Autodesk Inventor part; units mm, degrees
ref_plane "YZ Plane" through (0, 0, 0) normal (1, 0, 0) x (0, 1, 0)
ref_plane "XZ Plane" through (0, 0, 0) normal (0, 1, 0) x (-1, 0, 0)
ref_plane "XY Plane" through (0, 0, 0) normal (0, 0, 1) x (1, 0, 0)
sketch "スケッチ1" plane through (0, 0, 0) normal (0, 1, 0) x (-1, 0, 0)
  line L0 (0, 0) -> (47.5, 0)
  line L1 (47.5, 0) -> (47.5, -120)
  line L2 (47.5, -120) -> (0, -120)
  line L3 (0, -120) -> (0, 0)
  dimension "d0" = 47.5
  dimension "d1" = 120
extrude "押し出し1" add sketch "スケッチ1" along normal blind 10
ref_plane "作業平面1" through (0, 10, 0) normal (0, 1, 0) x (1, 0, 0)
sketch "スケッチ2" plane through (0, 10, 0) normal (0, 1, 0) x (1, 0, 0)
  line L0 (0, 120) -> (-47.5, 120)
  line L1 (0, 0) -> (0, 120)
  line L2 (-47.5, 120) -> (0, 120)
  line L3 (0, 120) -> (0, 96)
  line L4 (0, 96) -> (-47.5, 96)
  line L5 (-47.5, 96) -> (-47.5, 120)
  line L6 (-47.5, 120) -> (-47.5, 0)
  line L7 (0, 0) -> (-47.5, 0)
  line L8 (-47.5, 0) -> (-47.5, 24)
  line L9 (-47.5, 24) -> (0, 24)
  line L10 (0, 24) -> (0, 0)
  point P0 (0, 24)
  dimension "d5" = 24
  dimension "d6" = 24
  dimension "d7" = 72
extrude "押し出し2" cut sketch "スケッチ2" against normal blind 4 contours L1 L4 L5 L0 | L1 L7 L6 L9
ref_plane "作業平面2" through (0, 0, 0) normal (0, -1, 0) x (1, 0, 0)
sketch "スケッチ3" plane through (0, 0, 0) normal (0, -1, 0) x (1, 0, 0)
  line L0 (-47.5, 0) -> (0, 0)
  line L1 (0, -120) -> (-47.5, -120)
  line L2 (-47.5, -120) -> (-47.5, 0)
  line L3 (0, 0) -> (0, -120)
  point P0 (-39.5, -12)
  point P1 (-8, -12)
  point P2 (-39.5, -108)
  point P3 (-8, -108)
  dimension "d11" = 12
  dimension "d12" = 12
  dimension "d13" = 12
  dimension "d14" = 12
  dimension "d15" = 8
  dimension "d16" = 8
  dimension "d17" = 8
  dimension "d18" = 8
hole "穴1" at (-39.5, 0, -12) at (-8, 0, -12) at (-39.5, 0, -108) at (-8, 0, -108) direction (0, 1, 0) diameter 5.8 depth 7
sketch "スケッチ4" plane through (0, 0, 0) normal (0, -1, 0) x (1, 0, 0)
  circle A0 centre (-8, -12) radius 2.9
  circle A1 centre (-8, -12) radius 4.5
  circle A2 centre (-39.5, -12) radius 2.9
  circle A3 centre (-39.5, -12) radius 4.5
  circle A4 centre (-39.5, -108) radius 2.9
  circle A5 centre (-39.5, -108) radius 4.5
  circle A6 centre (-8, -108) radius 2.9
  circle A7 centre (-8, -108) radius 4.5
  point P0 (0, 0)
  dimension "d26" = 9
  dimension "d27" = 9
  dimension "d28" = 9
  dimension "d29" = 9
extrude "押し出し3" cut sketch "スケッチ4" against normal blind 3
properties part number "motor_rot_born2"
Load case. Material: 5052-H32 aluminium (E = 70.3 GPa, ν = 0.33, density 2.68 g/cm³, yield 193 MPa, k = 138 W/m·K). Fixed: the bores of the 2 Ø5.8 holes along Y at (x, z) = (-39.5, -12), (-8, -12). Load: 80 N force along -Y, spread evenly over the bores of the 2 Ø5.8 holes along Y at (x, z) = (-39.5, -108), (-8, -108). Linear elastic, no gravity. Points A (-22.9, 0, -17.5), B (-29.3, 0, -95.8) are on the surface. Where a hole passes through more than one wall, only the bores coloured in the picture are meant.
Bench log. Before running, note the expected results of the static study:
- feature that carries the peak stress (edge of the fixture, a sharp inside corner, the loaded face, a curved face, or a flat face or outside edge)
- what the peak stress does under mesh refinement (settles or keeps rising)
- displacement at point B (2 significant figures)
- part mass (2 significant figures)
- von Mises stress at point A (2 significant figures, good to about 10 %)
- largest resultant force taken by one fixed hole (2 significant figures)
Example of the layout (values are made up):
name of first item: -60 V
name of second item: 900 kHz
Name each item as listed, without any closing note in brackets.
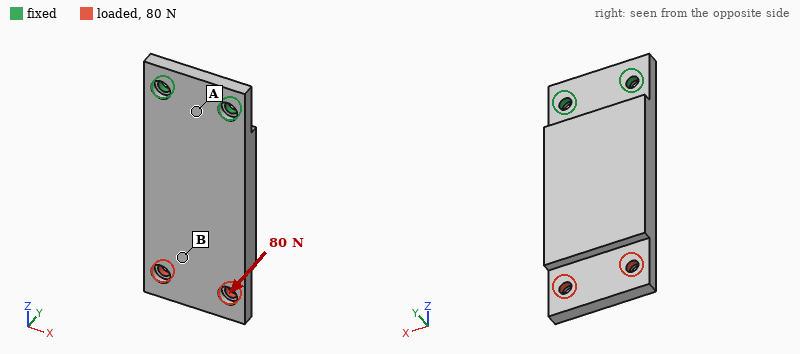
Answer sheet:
feature that carries the peak stress: edge of the fixture
what the peak stress does under mesh refinement: keeps rising
displacement at point B: 0.25 mm
part mass: 130 g
von Mises stress at point A: 21 MPa
largest resultant force taken by one fixed hole: 52 N
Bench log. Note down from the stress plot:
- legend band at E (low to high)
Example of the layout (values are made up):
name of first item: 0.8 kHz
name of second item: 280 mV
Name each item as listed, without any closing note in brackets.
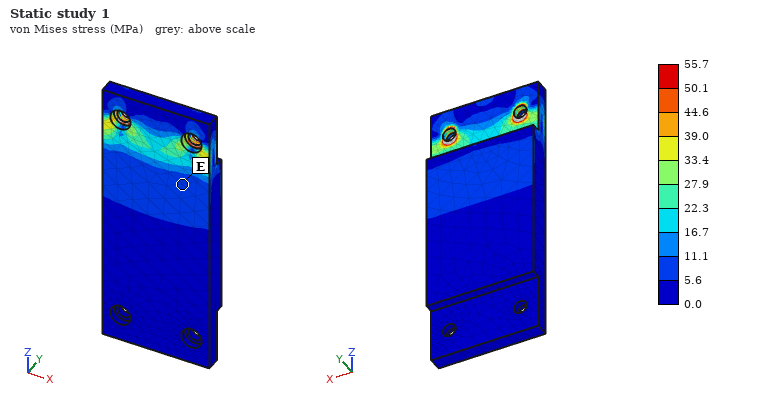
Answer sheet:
legend band at E: 5.6 to 11.1 MPa
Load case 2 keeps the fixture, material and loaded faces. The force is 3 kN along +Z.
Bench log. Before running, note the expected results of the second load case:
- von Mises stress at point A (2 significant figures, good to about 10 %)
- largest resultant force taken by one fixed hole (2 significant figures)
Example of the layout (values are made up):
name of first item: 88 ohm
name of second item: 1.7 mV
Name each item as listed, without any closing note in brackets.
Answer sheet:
von Mises stress at point A: 5.4 MPa
largest resultant force taken by one fixed hole: 1.5 kN
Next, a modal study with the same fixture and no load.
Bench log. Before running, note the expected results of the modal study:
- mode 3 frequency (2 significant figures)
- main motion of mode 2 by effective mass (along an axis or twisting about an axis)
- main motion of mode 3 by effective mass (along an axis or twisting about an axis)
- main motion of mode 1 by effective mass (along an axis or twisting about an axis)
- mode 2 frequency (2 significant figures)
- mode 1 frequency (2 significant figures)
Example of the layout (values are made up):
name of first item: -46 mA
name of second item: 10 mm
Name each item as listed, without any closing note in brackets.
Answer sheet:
mode 3 frequency: 2800 Hz
main motion of mode 2 by effective mass: along X
main motion of mode 3 by effective mass: twisting about Z
main motion of mode 1 by effective mass: along Y
mode 2 frequency: 2600 Hz
mode 1 frequency: 420 Hz
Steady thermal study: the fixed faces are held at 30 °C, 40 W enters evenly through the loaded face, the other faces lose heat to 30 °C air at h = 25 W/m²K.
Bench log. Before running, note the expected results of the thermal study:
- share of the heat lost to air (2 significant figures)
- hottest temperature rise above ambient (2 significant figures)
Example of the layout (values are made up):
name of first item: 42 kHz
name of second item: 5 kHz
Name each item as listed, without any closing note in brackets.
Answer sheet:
share of the heat lost to air: 28 %
hottest temperature rise above ambient: 69 K
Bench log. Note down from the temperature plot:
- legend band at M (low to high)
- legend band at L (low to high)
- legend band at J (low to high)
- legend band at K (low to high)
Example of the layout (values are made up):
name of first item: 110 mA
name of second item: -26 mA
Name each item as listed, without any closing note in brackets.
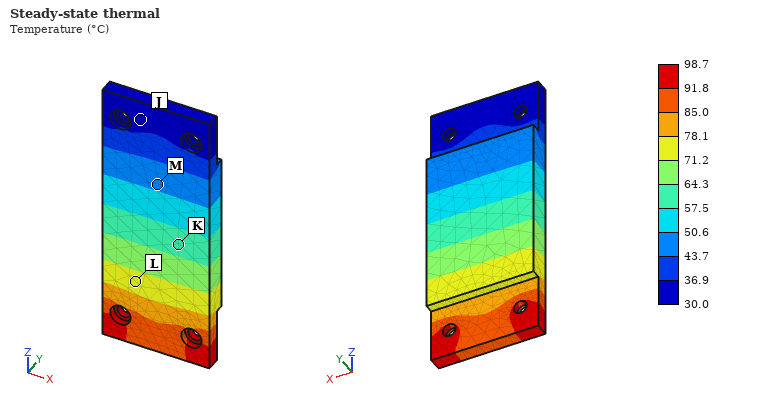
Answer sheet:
legend band at M: 43.7 to 50.6 °C
legend band at L: 71.2 to 78.1 °C
legend band at J: 30.0 to 36.9 °C
legend band at K: 57.5 to 64.3 °C
